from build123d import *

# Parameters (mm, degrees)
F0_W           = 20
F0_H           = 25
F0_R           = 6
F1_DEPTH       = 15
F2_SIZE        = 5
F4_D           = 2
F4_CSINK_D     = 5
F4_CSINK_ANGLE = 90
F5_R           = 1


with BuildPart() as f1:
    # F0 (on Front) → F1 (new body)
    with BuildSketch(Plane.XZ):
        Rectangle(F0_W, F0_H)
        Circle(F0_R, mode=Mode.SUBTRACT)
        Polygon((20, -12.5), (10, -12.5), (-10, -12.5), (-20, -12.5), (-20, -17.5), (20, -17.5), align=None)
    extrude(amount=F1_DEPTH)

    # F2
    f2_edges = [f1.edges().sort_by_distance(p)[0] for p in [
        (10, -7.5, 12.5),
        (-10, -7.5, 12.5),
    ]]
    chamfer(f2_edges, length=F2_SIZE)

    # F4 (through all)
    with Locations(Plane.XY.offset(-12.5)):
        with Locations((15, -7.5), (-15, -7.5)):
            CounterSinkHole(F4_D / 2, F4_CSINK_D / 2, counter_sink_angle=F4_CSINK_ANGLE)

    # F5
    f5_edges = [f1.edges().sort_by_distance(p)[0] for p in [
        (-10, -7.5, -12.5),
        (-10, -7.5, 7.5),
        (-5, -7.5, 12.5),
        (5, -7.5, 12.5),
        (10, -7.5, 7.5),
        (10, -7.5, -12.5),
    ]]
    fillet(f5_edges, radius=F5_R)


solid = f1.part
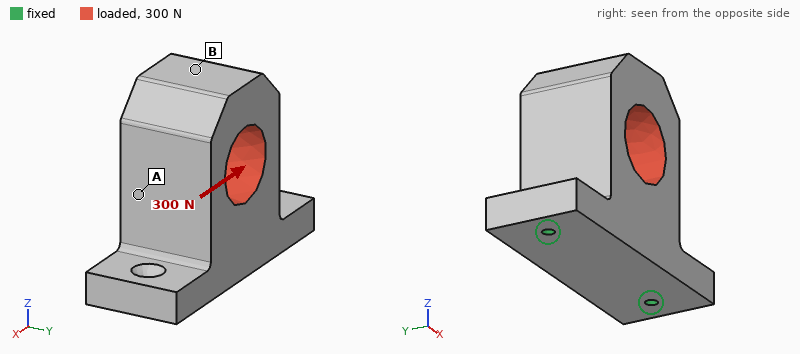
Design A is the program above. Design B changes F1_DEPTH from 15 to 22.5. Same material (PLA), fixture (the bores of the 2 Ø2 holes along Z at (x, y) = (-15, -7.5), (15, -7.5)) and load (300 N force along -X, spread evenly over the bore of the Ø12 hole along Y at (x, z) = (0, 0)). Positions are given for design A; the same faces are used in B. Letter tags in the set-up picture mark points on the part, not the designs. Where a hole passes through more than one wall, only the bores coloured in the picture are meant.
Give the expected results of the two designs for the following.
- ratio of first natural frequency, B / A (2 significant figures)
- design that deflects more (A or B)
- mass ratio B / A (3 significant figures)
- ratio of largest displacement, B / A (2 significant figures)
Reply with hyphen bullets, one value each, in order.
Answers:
- 0.81
- A
- 1.50
- 0.83
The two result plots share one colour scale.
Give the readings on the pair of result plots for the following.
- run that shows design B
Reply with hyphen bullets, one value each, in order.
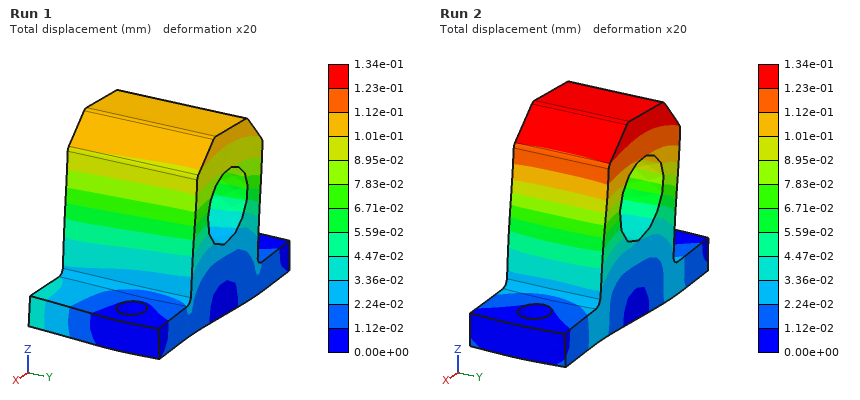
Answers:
- Run 1
